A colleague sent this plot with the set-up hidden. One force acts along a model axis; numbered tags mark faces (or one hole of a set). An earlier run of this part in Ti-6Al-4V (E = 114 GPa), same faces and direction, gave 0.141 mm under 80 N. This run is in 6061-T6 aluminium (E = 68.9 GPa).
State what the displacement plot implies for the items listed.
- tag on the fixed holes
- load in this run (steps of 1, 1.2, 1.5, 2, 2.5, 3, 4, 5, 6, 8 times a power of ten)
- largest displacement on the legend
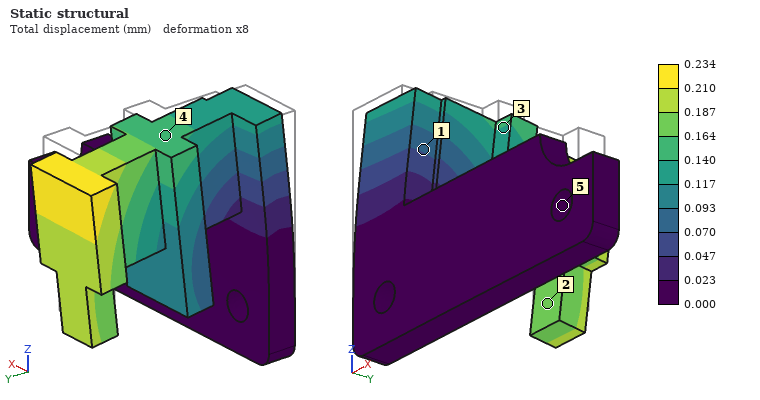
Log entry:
5
80 N
0.234 mm
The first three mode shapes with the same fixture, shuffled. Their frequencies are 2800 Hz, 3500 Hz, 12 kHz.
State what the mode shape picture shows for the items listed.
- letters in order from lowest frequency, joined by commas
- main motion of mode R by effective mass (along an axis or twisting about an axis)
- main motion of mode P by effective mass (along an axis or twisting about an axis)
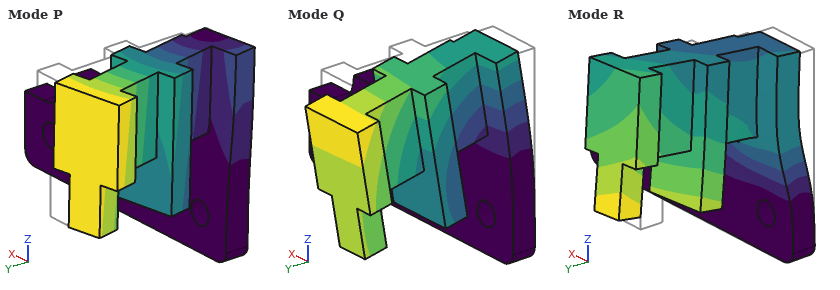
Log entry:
Q, P, R
along Y
along X
